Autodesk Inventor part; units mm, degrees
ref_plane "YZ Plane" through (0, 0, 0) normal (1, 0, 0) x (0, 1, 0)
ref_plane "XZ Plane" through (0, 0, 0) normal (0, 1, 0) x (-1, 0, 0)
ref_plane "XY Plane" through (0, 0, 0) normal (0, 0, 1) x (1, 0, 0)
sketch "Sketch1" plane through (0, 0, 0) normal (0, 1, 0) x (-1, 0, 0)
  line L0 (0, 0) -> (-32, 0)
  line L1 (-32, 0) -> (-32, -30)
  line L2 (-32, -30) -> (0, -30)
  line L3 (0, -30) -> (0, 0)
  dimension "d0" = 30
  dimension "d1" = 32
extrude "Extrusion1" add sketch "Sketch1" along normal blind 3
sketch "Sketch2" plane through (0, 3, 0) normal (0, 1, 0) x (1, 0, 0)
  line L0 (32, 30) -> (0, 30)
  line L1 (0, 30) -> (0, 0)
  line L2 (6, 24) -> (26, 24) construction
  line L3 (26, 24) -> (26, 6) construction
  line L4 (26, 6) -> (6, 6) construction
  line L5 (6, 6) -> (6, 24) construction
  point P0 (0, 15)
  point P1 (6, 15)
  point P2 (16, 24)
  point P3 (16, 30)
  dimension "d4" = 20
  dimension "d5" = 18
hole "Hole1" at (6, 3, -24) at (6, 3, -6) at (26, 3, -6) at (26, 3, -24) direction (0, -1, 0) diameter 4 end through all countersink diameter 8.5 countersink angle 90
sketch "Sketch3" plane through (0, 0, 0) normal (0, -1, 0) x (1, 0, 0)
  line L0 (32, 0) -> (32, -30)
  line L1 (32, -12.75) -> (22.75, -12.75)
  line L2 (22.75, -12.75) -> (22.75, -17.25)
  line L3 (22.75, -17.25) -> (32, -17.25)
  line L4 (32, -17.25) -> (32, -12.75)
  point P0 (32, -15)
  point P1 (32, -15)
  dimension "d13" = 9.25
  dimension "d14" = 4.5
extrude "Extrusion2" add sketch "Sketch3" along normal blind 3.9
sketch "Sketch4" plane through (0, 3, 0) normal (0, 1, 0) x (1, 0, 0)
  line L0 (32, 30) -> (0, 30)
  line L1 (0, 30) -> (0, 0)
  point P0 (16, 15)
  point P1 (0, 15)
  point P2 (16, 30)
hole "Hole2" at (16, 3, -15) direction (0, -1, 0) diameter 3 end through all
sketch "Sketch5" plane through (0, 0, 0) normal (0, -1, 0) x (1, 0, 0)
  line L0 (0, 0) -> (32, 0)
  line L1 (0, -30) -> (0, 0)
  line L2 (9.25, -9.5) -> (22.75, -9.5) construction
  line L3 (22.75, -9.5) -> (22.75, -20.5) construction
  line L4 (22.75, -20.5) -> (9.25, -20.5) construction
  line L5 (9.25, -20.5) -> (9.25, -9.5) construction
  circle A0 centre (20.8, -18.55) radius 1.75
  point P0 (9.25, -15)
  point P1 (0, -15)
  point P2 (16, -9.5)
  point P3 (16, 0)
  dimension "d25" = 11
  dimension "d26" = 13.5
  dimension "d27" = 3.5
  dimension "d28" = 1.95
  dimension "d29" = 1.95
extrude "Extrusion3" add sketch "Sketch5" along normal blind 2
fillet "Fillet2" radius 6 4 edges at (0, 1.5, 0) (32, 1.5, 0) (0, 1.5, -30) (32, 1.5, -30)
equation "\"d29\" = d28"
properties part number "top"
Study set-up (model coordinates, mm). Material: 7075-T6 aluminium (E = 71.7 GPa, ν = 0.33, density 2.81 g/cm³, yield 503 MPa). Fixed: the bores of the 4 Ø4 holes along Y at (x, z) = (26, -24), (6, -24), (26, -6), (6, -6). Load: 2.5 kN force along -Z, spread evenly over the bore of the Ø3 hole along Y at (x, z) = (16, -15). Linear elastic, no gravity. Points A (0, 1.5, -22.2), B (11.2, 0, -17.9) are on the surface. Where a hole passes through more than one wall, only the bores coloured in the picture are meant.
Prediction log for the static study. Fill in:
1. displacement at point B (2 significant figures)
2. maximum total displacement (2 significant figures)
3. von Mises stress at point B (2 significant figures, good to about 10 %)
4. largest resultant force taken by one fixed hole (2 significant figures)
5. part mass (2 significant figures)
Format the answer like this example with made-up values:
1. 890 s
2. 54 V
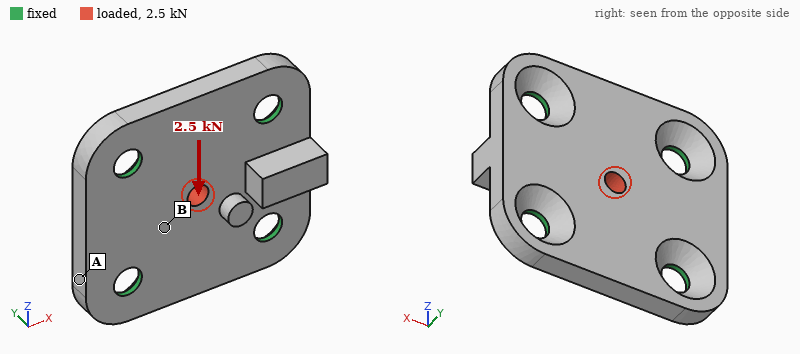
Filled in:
1. 5.5 µm
2. 11 µm
3. 37 MPa
4. 680 N
5. 7.4 g
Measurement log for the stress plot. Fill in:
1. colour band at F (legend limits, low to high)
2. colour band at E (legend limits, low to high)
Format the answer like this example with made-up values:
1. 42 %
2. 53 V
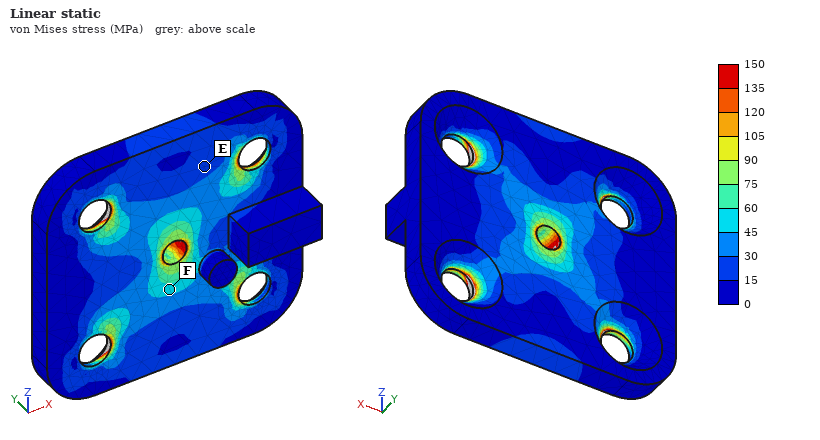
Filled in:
1. 45 to 60 MPa
2. 15 to 30 MPa
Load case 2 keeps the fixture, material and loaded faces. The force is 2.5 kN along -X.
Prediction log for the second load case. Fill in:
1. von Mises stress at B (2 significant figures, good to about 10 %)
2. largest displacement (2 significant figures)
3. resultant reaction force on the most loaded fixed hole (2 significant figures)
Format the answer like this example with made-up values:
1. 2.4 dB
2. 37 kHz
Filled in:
1. 45 MPa
2. 10 µm
3. 660 N
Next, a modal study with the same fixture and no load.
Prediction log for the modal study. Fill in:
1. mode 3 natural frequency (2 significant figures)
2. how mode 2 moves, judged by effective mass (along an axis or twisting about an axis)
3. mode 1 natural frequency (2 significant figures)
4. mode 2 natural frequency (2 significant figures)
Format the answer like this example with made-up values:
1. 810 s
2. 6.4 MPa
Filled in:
1. 28 kHz
2. along Y
3. 24 kHz
4. 26 kHz
